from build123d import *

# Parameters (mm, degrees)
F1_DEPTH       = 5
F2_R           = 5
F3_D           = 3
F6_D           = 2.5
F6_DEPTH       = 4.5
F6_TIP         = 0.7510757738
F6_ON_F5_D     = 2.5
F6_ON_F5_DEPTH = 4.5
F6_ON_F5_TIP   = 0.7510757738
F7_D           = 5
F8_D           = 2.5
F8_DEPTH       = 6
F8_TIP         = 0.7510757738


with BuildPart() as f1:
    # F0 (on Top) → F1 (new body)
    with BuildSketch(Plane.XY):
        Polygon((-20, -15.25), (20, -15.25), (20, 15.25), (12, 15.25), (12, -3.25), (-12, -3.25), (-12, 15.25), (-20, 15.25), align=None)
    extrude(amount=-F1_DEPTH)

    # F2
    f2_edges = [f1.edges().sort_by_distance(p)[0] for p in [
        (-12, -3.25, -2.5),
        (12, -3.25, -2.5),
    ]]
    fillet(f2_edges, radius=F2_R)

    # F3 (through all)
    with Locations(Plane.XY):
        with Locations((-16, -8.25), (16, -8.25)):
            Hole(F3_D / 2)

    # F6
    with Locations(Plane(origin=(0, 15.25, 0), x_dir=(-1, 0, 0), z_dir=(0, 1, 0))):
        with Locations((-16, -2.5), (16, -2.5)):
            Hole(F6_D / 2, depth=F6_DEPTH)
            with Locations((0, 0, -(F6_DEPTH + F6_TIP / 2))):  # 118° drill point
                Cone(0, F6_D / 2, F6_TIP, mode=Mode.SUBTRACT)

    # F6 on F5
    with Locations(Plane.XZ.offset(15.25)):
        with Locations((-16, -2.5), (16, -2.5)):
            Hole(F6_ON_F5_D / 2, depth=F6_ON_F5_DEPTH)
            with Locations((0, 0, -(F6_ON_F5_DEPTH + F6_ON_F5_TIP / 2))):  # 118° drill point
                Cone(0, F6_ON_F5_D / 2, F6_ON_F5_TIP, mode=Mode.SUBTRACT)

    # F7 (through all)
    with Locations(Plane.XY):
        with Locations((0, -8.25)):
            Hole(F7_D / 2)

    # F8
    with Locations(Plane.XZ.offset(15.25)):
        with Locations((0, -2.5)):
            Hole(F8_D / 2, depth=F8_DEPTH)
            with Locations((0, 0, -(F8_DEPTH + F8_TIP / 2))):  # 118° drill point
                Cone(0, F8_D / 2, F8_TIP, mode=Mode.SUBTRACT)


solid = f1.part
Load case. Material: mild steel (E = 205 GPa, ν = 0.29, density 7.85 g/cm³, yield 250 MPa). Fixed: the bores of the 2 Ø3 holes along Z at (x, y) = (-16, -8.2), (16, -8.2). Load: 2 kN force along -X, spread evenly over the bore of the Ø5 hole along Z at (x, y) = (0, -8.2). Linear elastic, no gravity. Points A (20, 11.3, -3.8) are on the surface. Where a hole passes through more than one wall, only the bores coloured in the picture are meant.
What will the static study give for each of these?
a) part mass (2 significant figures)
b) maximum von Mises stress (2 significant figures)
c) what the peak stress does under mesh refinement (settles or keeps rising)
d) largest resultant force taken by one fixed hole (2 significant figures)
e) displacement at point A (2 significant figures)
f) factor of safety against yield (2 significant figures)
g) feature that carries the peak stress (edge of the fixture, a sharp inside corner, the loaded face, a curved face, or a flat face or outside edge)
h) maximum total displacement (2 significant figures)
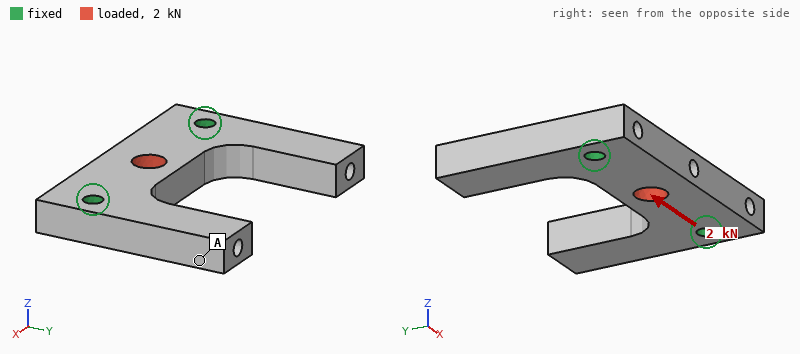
29 g
61 MPa
settles
1.0 kN
1.1 µm
4.1
the loaded face
1.7 µm
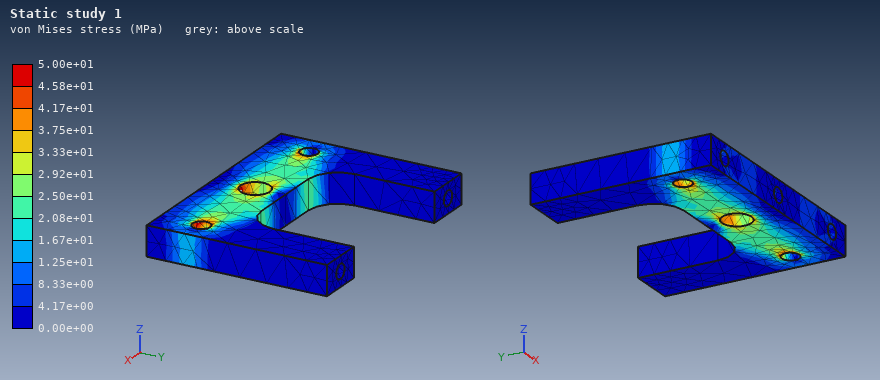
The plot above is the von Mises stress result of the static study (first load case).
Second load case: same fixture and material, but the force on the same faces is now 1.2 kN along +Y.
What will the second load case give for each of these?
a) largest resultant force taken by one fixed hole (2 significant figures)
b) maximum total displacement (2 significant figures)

610 N
7.1 µm
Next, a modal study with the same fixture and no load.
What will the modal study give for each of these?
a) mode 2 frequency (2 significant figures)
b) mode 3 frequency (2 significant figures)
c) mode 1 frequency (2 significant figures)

8500 Hz
13 kHz
8300 Hz
